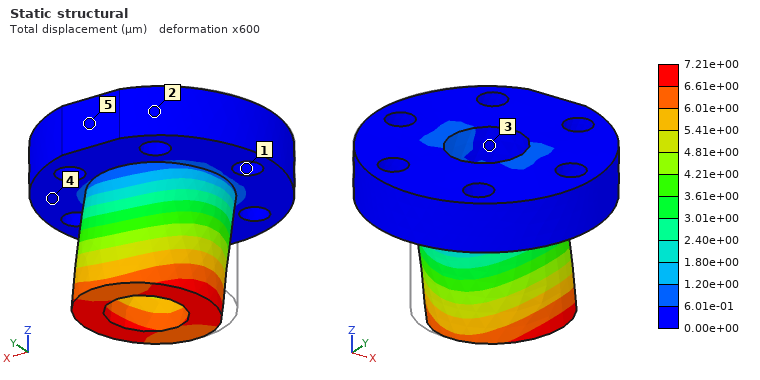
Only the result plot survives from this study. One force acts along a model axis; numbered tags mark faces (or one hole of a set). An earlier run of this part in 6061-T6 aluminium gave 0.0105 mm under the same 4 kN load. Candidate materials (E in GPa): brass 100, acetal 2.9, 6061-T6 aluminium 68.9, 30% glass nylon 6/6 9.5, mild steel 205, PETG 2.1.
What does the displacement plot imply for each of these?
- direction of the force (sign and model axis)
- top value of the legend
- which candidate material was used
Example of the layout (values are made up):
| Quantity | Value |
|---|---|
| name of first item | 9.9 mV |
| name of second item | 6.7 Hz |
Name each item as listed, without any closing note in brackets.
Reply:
| Quantity | Value |
|---|---|
| direction of the force | +X |
| top value of the legend | 7.21e+00 µm |
| which candidate material was used | brass |
